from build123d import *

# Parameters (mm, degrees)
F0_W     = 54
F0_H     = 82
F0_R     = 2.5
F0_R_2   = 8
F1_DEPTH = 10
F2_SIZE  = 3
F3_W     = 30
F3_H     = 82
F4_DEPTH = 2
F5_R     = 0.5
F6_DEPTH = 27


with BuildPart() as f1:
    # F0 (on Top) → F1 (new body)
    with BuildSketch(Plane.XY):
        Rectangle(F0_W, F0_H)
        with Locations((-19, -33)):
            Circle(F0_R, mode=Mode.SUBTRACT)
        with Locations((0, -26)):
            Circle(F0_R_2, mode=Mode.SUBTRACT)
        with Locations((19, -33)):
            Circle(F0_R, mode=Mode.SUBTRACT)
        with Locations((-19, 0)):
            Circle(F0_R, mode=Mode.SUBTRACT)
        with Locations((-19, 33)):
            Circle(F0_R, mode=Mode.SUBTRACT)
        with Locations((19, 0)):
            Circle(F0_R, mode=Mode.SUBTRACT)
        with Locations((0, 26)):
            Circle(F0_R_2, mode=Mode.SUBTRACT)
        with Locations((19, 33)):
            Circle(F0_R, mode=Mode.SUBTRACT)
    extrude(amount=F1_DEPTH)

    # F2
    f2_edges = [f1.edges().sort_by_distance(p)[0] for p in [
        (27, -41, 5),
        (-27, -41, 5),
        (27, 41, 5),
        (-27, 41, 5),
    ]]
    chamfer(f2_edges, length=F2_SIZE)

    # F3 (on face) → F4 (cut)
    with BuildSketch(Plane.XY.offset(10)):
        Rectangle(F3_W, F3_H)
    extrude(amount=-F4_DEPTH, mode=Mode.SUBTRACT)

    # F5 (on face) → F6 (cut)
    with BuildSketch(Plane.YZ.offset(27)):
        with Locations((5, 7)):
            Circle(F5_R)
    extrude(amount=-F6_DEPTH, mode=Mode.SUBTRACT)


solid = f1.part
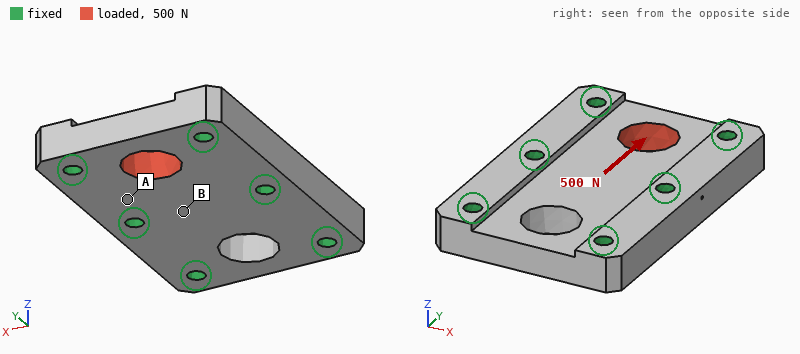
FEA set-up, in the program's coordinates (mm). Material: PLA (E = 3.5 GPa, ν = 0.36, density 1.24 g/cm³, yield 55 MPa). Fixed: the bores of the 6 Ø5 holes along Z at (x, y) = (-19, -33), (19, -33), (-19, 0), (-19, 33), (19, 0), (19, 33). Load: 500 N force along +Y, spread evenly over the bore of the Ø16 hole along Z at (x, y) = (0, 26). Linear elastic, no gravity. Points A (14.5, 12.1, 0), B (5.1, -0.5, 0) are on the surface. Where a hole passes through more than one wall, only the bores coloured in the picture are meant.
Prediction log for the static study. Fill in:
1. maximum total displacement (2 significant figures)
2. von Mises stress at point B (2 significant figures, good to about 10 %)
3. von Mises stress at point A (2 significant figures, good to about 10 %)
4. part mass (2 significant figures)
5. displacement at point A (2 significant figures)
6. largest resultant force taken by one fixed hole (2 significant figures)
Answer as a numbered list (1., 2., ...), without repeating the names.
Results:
1. 19 µm
2. 0.43 MPa
3. 1.0 MPa
4. 43 g
5. 2.9 µm
6. 140 N
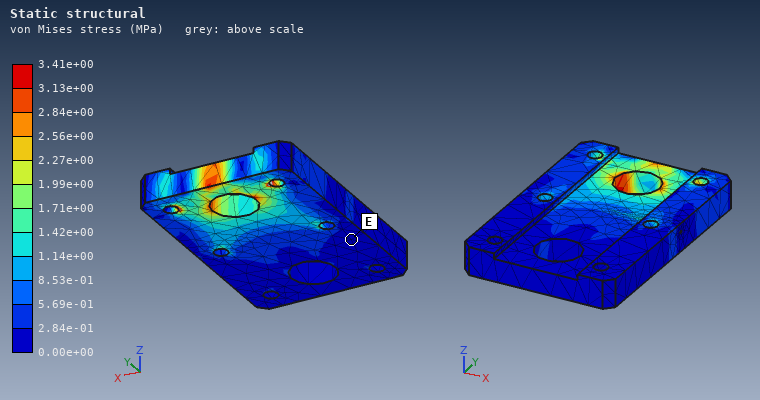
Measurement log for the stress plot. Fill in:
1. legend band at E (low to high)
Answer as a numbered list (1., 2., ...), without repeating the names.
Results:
1. 0.00e+00 to 2.84e-01 MPa
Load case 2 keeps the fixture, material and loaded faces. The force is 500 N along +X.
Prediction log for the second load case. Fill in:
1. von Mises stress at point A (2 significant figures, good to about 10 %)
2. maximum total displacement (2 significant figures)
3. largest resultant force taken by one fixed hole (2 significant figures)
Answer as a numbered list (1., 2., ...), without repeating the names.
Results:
1. 0.77 MPa
2. 7.6 µm
3. 180 N
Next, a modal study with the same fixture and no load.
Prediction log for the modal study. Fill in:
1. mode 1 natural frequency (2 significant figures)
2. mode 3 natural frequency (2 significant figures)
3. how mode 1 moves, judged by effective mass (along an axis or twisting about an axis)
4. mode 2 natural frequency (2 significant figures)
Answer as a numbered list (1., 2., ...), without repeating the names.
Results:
1. 7200 Hz
2. 9700 Hz
3. along Z
4. 8100 Hz
